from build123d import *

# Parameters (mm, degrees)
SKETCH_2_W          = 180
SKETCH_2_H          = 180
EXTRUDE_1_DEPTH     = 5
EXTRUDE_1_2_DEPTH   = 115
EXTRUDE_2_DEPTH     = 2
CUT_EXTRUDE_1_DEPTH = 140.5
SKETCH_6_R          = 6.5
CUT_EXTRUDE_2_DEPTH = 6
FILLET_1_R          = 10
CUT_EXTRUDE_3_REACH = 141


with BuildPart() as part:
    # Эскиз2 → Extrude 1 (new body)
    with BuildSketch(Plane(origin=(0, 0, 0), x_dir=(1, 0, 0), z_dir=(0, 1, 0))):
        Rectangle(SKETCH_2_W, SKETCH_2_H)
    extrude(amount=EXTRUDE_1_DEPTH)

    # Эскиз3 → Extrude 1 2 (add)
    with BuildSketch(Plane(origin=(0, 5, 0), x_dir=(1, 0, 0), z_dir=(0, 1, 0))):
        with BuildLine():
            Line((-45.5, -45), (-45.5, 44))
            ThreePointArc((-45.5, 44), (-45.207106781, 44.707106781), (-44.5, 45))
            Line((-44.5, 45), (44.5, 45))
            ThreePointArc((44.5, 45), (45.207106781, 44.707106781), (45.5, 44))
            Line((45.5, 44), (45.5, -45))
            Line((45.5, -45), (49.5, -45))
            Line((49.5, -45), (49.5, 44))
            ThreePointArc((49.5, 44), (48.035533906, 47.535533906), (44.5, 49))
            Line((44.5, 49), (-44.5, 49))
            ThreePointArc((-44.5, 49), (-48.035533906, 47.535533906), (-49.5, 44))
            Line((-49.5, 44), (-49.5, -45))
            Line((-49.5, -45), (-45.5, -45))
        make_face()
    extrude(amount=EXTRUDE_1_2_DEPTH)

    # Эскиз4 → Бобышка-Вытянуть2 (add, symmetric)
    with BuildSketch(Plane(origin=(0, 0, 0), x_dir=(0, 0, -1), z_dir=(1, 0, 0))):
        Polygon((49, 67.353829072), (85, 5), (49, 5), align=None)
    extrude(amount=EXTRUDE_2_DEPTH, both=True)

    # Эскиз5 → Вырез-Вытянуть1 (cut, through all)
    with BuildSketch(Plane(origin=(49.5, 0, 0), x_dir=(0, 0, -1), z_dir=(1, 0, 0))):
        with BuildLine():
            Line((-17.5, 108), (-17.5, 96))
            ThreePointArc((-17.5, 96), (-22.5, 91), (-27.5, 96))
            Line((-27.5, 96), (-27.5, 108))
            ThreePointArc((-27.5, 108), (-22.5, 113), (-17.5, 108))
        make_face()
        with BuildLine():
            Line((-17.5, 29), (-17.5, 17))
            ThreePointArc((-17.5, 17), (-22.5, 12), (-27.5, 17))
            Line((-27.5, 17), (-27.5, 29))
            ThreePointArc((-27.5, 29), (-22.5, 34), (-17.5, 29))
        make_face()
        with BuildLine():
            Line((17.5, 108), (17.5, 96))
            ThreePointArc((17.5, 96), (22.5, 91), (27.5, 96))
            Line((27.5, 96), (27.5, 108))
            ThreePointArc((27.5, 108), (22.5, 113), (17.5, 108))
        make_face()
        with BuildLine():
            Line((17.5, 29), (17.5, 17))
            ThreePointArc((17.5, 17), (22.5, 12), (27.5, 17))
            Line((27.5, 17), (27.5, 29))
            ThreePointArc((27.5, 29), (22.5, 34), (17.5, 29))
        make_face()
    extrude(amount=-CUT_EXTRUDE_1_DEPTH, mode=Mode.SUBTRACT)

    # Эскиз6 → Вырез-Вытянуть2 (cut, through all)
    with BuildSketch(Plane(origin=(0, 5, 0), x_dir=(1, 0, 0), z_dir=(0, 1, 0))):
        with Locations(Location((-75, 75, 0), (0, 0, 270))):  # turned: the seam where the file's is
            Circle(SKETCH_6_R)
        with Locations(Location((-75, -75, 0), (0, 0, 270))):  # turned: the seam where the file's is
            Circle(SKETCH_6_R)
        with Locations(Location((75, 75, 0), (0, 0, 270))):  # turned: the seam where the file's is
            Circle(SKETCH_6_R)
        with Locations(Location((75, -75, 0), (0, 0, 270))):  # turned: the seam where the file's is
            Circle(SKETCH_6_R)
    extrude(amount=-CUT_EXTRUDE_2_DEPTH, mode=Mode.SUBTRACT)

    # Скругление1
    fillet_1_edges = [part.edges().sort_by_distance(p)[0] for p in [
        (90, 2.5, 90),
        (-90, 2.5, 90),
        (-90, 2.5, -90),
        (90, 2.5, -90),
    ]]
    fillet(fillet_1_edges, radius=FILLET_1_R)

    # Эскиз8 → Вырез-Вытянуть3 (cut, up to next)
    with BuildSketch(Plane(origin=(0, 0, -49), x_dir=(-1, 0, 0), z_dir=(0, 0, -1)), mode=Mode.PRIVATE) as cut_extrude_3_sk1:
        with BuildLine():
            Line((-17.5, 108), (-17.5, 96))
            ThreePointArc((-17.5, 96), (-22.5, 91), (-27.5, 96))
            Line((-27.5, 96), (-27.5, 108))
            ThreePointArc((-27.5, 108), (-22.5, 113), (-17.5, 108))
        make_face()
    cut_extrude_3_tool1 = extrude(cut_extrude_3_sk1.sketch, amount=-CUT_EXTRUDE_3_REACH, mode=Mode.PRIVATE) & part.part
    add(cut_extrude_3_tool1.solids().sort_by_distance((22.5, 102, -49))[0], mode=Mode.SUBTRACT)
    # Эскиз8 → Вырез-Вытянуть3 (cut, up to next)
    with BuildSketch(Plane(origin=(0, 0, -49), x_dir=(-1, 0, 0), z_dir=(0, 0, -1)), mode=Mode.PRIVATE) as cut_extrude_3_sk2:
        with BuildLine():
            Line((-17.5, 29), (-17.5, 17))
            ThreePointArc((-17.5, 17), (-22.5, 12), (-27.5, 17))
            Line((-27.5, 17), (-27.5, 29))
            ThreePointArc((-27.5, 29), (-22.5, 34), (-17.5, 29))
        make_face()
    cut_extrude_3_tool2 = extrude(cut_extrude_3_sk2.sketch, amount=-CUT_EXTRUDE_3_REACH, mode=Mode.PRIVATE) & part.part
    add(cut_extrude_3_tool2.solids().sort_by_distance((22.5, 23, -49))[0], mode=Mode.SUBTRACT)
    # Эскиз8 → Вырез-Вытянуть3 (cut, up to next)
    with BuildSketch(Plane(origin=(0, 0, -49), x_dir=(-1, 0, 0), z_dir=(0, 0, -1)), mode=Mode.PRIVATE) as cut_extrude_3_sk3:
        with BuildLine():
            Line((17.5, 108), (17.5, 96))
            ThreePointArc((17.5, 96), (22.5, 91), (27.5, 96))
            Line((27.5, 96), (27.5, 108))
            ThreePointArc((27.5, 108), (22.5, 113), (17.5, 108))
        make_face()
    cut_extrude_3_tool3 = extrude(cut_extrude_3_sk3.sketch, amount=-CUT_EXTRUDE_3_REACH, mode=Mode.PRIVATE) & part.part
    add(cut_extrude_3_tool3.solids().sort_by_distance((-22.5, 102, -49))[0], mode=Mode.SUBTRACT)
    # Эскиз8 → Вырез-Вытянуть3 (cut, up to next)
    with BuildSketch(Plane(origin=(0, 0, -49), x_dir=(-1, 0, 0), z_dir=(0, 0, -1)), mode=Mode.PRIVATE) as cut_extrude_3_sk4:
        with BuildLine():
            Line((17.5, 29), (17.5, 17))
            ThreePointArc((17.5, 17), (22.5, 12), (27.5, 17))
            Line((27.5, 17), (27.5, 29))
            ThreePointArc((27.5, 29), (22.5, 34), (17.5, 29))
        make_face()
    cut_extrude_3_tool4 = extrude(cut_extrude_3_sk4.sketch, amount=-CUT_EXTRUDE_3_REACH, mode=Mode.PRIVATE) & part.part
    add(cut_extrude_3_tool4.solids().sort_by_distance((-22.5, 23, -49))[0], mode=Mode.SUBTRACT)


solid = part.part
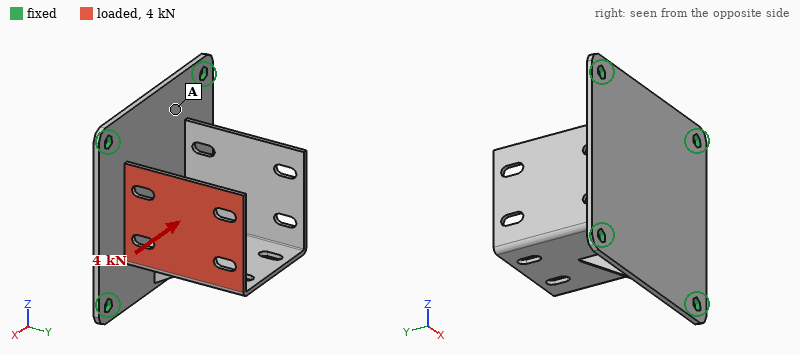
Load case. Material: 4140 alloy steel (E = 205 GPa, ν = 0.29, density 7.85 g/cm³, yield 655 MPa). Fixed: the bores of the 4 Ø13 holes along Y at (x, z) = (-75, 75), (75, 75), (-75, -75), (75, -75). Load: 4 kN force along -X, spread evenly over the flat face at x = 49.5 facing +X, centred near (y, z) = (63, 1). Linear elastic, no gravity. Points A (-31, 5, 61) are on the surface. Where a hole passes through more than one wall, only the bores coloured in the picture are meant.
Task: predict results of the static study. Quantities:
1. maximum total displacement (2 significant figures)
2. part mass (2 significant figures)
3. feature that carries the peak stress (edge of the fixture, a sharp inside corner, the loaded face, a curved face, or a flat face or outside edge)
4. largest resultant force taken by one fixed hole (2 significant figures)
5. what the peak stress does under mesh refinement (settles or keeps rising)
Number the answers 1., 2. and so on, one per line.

1. 2.8 mm
2. 2.2 kg
3. a sharp inside corner
4. 2.2 kN
5. keeps rising
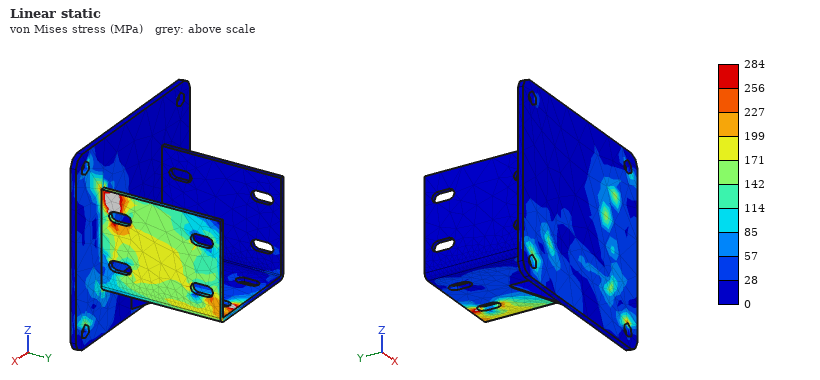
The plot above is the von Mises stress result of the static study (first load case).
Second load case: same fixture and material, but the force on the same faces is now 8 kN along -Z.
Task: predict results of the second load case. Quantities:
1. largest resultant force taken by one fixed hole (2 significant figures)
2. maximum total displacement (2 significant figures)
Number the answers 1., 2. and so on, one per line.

1. 4.7 kN
2. 0.76 mm
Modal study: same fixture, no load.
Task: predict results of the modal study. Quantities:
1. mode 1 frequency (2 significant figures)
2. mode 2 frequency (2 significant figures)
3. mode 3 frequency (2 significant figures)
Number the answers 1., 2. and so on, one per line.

1. 500 Hz
2. 500 Hz
3. 880 Hz
